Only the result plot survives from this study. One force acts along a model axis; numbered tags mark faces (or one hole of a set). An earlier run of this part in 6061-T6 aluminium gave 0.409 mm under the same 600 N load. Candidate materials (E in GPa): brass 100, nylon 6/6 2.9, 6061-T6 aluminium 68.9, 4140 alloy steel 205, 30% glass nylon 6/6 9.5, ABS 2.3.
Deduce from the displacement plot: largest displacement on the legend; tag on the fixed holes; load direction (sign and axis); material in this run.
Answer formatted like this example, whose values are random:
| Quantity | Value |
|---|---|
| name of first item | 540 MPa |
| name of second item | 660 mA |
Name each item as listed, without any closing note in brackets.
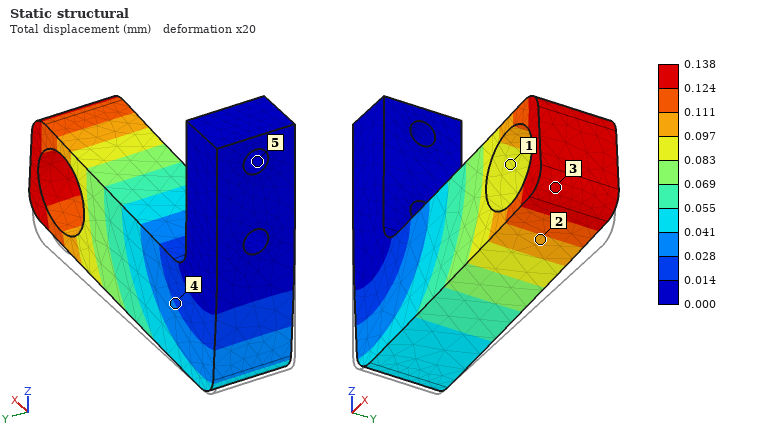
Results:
| Quantity | Value |
|---|---|
| largest displacement on the legend | 0.138 mm |
| tag on the fixed holes | 5 |
| load direction | +Z |
| material in this run | 4140 alloy steel |
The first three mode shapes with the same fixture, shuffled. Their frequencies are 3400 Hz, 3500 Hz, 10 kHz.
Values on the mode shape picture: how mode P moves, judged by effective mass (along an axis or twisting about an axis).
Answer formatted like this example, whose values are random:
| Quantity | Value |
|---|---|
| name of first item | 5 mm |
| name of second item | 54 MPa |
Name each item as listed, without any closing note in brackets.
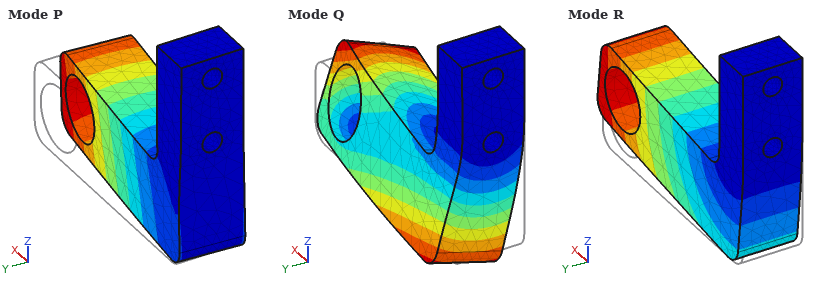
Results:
| Quantity | Value |
|---|---|
| how mode P moves, judged by effective mass | along Y |
